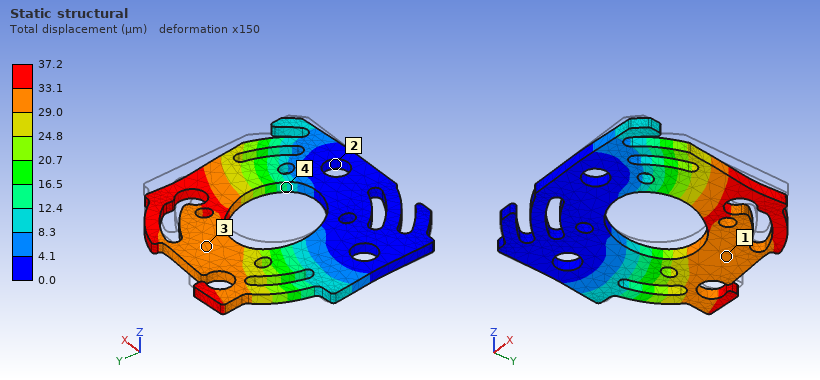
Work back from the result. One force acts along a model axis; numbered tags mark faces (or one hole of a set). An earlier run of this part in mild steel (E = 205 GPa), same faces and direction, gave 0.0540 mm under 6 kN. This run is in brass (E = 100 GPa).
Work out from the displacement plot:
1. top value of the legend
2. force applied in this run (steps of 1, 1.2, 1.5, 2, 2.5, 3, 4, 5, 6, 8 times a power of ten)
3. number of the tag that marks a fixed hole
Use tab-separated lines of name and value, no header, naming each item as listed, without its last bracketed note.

top value of the legend	37.2 µm
force applied in this run	2 kN
number of the tag that marks a fixed hole	2
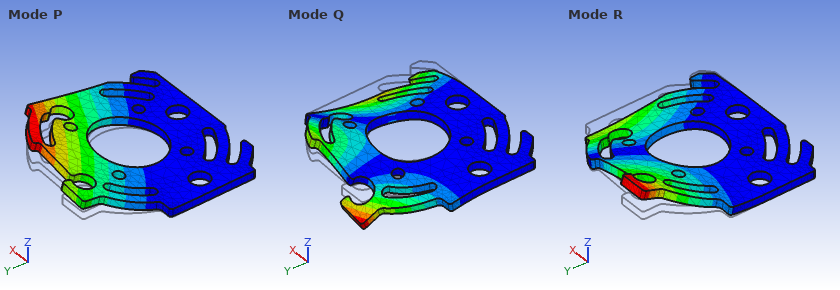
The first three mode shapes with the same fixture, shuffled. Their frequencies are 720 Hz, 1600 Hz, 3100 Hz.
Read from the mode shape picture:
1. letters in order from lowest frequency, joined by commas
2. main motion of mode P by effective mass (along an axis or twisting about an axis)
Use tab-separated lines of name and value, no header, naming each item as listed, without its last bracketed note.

letters in order from lowest frequency, joined by commas	P, R, Q
main motion of mode P by effective mass	along Z
